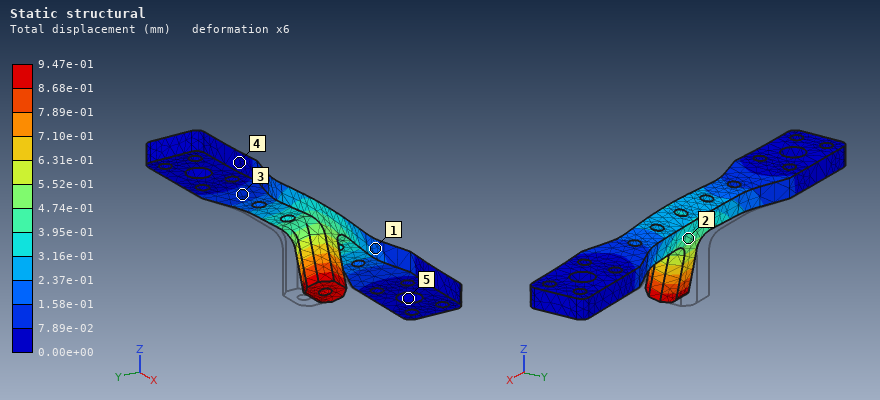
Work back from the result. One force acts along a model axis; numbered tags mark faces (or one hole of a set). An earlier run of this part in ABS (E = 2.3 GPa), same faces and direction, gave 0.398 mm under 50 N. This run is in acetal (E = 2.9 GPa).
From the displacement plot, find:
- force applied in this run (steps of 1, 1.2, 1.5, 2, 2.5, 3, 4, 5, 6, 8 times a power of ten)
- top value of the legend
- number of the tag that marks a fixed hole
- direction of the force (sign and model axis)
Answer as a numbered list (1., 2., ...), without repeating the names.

1. 150 N
2. 9.47e-01 mm
3. 5
4. -Y
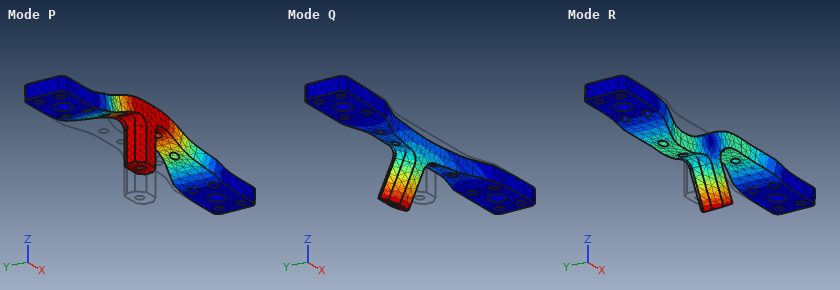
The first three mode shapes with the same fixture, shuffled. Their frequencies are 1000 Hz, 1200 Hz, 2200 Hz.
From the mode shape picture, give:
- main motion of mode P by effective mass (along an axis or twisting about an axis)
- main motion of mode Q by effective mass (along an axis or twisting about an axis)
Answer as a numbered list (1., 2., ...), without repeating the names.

1. along Z
2. along Y
